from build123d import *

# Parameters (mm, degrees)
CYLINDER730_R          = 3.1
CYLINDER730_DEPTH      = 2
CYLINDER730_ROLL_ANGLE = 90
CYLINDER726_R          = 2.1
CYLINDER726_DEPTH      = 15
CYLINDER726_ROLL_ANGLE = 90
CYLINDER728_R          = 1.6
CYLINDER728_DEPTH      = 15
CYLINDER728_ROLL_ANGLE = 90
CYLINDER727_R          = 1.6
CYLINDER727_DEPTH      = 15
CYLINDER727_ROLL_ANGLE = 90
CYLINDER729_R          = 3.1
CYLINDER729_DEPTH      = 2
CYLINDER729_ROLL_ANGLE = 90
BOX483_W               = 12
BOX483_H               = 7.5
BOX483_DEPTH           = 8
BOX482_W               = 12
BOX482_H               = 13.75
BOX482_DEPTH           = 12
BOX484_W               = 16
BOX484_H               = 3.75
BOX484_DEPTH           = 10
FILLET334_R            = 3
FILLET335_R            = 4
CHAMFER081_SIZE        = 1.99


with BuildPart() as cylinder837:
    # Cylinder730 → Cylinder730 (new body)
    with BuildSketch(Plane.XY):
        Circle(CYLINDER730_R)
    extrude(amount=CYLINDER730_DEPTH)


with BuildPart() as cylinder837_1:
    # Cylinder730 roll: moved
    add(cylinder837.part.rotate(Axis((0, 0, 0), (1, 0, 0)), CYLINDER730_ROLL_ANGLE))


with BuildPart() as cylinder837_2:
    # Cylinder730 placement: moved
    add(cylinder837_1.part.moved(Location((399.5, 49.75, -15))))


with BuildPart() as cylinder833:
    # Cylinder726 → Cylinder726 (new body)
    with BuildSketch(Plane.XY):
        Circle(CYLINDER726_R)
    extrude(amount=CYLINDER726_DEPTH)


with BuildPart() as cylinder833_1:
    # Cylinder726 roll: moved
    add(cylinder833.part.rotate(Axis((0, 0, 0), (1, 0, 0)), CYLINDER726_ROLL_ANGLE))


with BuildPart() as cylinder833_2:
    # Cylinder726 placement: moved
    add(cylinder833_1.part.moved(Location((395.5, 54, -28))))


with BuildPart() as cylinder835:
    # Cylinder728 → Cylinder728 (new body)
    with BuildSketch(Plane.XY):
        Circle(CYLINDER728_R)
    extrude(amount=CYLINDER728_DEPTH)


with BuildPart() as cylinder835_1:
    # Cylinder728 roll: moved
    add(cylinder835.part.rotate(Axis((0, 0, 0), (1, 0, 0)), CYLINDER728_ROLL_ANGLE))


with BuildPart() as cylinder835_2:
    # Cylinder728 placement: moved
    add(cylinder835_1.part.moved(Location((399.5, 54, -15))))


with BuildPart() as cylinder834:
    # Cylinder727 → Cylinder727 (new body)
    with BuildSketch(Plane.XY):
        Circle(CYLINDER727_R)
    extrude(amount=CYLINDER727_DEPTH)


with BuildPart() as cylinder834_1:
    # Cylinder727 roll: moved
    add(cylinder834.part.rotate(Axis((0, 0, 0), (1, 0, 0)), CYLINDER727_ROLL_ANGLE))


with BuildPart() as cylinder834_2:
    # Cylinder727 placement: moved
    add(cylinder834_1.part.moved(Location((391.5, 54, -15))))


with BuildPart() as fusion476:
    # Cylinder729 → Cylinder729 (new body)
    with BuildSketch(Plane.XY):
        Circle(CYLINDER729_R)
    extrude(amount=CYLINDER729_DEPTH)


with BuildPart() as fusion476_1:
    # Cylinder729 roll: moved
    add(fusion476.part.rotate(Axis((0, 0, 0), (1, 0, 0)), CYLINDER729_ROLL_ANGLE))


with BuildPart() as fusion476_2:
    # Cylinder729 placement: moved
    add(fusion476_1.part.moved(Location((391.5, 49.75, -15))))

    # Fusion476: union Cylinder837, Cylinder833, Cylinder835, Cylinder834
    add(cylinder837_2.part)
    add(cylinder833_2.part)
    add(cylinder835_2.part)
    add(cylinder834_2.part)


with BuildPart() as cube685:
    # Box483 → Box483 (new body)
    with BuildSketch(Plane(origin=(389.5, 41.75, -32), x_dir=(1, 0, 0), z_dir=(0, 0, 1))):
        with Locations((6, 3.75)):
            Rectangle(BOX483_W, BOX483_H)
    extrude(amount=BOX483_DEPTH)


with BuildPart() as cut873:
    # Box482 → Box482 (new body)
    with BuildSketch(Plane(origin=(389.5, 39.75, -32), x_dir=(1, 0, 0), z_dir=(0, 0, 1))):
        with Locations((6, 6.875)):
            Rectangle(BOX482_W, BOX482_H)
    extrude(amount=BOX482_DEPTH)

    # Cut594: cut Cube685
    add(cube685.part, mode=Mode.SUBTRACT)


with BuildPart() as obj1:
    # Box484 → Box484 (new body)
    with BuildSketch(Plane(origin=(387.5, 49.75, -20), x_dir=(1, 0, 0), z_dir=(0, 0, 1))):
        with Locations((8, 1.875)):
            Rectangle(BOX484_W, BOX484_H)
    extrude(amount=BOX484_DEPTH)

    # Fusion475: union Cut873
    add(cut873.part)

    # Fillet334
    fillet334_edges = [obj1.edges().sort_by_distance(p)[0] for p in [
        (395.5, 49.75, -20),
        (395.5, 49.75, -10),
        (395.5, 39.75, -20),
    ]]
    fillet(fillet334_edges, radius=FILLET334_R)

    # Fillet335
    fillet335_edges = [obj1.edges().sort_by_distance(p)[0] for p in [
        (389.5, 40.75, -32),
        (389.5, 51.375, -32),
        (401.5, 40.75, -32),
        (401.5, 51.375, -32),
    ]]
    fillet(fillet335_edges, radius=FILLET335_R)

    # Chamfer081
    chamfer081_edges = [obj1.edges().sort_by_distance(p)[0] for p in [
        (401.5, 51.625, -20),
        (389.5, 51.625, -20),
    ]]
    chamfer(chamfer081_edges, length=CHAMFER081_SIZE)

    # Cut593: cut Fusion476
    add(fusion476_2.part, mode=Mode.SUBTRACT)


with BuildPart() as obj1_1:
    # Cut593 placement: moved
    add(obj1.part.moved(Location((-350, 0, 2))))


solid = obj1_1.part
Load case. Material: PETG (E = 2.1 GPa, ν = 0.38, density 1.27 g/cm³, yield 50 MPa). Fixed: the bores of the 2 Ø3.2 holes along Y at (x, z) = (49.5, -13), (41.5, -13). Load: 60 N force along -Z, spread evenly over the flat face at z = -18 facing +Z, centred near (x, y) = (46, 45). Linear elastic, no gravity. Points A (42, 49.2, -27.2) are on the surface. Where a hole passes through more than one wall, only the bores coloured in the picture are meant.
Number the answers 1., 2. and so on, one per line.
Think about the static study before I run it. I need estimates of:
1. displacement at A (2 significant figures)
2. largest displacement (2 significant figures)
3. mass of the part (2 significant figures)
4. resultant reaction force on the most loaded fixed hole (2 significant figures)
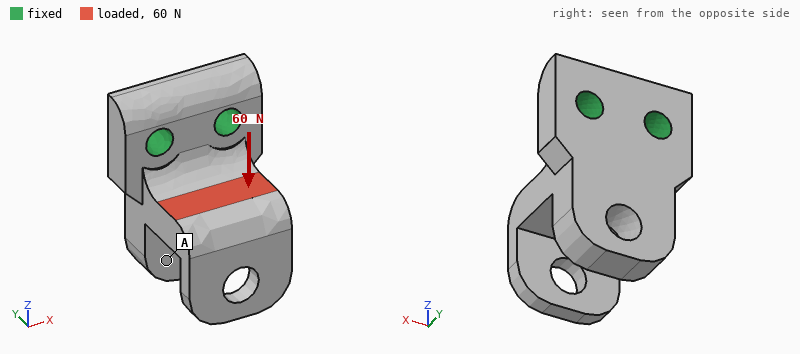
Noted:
1. 0.14 mm
2. 0.29 mm
3. 2.1 g
4. 32 N
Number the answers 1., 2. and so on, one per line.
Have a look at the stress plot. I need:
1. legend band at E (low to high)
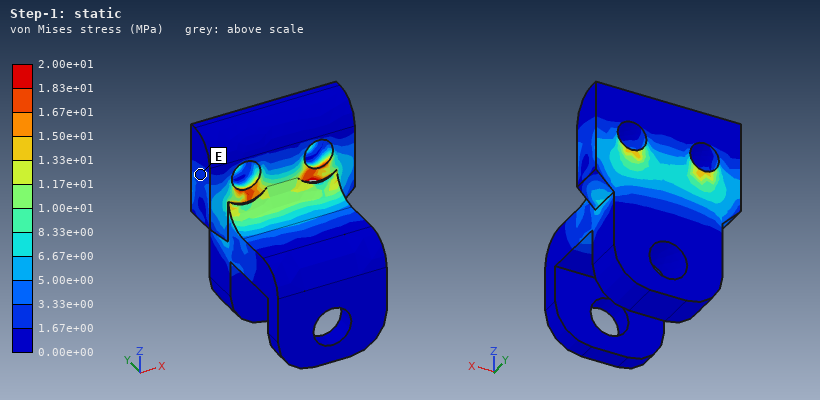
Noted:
1. 1.67e+00 to 3.33e+00 MPa
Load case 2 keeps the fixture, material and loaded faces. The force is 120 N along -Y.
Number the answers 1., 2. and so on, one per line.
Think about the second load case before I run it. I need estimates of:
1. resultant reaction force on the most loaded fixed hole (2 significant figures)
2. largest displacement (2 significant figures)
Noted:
1. 60 N
2. 0.13 mm
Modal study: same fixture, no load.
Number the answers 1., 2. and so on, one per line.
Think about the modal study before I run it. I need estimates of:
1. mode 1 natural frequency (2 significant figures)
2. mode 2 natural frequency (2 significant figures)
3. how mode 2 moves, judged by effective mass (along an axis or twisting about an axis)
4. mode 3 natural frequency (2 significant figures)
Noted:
1. 2300 Hz
2. 5000 Hz
3. along X
4. 5300 Hz
